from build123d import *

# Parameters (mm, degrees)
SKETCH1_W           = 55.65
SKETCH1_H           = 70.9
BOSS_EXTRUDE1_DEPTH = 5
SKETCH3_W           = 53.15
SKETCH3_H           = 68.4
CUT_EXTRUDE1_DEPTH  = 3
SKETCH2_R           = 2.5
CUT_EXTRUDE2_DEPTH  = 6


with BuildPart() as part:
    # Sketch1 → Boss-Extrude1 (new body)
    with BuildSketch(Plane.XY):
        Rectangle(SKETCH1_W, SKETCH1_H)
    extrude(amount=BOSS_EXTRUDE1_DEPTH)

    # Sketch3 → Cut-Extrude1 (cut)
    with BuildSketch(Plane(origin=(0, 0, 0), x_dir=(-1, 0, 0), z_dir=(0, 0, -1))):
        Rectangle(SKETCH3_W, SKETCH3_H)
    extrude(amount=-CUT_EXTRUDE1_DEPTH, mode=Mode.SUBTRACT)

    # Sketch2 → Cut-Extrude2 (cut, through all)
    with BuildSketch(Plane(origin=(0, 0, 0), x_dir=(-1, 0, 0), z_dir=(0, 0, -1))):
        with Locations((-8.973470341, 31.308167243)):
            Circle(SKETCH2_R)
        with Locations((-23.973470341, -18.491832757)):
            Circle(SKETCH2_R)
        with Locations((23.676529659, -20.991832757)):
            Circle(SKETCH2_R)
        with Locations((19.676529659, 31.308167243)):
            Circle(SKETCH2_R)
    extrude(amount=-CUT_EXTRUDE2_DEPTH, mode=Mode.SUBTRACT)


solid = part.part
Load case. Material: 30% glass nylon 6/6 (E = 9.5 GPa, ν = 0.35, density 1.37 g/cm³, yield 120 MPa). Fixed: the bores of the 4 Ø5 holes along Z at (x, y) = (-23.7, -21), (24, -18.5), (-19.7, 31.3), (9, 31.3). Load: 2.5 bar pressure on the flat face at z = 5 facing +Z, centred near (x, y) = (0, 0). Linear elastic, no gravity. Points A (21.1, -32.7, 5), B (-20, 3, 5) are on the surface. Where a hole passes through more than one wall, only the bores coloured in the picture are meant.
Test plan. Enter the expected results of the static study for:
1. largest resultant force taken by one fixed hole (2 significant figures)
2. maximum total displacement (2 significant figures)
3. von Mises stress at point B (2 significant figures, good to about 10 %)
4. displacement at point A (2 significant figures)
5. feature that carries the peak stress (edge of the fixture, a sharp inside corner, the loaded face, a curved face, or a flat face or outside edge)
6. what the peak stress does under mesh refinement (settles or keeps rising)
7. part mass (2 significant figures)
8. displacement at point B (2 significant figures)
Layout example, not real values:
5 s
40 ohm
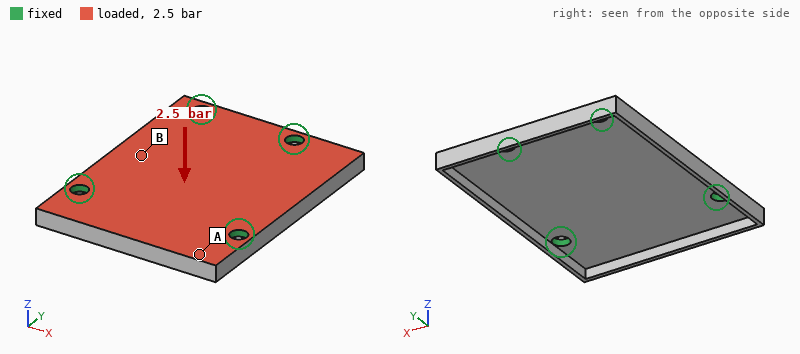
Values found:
290 N
0.81 mm
25 MPa
0.18 mm
edge of the fixture
keeps rising
12 g
0.48 mm
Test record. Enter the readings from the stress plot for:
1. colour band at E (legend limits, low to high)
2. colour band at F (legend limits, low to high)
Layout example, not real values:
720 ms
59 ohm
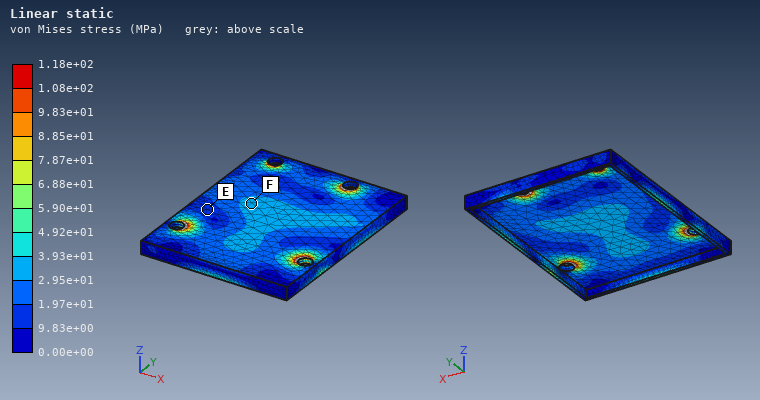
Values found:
9.83e+00 to 1.97e+01 MPa
2.95e+01 to 3.93e+01 MPa
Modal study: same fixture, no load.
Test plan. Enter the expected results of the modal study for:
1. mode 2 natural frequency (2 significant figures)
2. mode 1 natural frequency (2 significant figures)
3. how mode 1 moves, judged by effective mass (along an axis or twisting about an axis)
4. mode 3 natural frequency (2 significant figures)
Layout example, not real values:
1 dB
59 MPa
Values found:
2400 Hz
2100 Hz
along Z
2700 Hz
